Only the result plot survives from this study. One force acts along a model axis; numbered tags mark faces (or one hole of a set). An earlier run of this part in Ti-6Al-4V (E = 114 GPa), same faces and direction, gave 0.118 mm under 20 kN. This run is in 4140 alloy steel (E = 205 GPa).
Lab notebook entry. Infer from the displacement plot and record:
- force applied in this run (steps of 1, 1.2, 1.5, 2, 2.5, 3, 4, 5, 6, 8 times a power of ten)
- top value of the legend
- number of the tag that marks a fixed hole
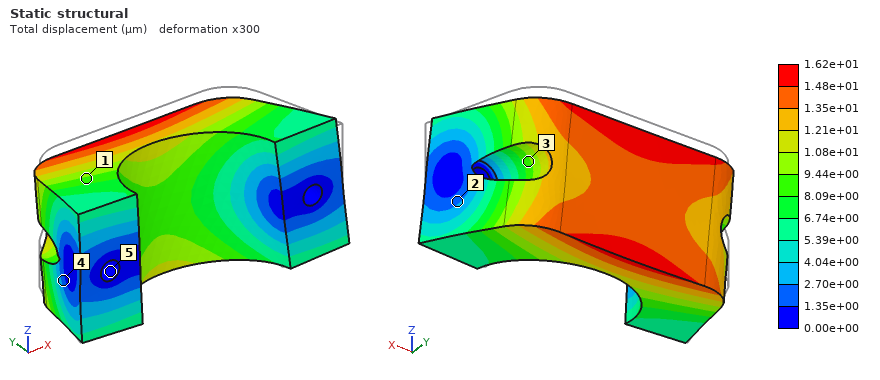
5 kN
1.62e+01 µm
5
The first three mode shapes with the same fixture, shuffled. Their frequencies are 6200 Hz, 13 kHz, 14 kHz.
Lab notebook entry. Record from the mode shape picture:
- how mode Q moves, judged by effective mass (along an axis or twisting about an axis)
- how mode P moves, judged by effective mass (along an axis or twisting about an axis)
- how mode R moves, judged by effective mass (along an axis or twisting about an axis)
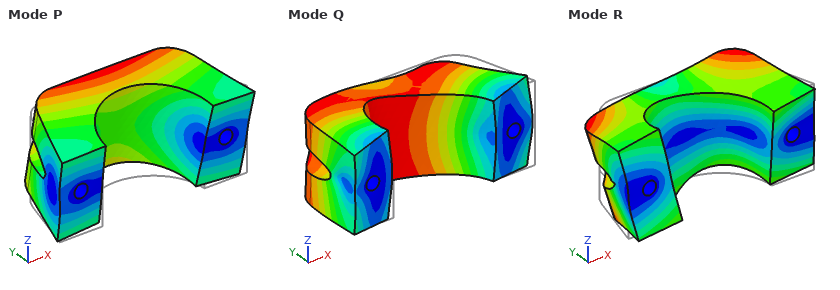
along X
along Z
twisting about Y
